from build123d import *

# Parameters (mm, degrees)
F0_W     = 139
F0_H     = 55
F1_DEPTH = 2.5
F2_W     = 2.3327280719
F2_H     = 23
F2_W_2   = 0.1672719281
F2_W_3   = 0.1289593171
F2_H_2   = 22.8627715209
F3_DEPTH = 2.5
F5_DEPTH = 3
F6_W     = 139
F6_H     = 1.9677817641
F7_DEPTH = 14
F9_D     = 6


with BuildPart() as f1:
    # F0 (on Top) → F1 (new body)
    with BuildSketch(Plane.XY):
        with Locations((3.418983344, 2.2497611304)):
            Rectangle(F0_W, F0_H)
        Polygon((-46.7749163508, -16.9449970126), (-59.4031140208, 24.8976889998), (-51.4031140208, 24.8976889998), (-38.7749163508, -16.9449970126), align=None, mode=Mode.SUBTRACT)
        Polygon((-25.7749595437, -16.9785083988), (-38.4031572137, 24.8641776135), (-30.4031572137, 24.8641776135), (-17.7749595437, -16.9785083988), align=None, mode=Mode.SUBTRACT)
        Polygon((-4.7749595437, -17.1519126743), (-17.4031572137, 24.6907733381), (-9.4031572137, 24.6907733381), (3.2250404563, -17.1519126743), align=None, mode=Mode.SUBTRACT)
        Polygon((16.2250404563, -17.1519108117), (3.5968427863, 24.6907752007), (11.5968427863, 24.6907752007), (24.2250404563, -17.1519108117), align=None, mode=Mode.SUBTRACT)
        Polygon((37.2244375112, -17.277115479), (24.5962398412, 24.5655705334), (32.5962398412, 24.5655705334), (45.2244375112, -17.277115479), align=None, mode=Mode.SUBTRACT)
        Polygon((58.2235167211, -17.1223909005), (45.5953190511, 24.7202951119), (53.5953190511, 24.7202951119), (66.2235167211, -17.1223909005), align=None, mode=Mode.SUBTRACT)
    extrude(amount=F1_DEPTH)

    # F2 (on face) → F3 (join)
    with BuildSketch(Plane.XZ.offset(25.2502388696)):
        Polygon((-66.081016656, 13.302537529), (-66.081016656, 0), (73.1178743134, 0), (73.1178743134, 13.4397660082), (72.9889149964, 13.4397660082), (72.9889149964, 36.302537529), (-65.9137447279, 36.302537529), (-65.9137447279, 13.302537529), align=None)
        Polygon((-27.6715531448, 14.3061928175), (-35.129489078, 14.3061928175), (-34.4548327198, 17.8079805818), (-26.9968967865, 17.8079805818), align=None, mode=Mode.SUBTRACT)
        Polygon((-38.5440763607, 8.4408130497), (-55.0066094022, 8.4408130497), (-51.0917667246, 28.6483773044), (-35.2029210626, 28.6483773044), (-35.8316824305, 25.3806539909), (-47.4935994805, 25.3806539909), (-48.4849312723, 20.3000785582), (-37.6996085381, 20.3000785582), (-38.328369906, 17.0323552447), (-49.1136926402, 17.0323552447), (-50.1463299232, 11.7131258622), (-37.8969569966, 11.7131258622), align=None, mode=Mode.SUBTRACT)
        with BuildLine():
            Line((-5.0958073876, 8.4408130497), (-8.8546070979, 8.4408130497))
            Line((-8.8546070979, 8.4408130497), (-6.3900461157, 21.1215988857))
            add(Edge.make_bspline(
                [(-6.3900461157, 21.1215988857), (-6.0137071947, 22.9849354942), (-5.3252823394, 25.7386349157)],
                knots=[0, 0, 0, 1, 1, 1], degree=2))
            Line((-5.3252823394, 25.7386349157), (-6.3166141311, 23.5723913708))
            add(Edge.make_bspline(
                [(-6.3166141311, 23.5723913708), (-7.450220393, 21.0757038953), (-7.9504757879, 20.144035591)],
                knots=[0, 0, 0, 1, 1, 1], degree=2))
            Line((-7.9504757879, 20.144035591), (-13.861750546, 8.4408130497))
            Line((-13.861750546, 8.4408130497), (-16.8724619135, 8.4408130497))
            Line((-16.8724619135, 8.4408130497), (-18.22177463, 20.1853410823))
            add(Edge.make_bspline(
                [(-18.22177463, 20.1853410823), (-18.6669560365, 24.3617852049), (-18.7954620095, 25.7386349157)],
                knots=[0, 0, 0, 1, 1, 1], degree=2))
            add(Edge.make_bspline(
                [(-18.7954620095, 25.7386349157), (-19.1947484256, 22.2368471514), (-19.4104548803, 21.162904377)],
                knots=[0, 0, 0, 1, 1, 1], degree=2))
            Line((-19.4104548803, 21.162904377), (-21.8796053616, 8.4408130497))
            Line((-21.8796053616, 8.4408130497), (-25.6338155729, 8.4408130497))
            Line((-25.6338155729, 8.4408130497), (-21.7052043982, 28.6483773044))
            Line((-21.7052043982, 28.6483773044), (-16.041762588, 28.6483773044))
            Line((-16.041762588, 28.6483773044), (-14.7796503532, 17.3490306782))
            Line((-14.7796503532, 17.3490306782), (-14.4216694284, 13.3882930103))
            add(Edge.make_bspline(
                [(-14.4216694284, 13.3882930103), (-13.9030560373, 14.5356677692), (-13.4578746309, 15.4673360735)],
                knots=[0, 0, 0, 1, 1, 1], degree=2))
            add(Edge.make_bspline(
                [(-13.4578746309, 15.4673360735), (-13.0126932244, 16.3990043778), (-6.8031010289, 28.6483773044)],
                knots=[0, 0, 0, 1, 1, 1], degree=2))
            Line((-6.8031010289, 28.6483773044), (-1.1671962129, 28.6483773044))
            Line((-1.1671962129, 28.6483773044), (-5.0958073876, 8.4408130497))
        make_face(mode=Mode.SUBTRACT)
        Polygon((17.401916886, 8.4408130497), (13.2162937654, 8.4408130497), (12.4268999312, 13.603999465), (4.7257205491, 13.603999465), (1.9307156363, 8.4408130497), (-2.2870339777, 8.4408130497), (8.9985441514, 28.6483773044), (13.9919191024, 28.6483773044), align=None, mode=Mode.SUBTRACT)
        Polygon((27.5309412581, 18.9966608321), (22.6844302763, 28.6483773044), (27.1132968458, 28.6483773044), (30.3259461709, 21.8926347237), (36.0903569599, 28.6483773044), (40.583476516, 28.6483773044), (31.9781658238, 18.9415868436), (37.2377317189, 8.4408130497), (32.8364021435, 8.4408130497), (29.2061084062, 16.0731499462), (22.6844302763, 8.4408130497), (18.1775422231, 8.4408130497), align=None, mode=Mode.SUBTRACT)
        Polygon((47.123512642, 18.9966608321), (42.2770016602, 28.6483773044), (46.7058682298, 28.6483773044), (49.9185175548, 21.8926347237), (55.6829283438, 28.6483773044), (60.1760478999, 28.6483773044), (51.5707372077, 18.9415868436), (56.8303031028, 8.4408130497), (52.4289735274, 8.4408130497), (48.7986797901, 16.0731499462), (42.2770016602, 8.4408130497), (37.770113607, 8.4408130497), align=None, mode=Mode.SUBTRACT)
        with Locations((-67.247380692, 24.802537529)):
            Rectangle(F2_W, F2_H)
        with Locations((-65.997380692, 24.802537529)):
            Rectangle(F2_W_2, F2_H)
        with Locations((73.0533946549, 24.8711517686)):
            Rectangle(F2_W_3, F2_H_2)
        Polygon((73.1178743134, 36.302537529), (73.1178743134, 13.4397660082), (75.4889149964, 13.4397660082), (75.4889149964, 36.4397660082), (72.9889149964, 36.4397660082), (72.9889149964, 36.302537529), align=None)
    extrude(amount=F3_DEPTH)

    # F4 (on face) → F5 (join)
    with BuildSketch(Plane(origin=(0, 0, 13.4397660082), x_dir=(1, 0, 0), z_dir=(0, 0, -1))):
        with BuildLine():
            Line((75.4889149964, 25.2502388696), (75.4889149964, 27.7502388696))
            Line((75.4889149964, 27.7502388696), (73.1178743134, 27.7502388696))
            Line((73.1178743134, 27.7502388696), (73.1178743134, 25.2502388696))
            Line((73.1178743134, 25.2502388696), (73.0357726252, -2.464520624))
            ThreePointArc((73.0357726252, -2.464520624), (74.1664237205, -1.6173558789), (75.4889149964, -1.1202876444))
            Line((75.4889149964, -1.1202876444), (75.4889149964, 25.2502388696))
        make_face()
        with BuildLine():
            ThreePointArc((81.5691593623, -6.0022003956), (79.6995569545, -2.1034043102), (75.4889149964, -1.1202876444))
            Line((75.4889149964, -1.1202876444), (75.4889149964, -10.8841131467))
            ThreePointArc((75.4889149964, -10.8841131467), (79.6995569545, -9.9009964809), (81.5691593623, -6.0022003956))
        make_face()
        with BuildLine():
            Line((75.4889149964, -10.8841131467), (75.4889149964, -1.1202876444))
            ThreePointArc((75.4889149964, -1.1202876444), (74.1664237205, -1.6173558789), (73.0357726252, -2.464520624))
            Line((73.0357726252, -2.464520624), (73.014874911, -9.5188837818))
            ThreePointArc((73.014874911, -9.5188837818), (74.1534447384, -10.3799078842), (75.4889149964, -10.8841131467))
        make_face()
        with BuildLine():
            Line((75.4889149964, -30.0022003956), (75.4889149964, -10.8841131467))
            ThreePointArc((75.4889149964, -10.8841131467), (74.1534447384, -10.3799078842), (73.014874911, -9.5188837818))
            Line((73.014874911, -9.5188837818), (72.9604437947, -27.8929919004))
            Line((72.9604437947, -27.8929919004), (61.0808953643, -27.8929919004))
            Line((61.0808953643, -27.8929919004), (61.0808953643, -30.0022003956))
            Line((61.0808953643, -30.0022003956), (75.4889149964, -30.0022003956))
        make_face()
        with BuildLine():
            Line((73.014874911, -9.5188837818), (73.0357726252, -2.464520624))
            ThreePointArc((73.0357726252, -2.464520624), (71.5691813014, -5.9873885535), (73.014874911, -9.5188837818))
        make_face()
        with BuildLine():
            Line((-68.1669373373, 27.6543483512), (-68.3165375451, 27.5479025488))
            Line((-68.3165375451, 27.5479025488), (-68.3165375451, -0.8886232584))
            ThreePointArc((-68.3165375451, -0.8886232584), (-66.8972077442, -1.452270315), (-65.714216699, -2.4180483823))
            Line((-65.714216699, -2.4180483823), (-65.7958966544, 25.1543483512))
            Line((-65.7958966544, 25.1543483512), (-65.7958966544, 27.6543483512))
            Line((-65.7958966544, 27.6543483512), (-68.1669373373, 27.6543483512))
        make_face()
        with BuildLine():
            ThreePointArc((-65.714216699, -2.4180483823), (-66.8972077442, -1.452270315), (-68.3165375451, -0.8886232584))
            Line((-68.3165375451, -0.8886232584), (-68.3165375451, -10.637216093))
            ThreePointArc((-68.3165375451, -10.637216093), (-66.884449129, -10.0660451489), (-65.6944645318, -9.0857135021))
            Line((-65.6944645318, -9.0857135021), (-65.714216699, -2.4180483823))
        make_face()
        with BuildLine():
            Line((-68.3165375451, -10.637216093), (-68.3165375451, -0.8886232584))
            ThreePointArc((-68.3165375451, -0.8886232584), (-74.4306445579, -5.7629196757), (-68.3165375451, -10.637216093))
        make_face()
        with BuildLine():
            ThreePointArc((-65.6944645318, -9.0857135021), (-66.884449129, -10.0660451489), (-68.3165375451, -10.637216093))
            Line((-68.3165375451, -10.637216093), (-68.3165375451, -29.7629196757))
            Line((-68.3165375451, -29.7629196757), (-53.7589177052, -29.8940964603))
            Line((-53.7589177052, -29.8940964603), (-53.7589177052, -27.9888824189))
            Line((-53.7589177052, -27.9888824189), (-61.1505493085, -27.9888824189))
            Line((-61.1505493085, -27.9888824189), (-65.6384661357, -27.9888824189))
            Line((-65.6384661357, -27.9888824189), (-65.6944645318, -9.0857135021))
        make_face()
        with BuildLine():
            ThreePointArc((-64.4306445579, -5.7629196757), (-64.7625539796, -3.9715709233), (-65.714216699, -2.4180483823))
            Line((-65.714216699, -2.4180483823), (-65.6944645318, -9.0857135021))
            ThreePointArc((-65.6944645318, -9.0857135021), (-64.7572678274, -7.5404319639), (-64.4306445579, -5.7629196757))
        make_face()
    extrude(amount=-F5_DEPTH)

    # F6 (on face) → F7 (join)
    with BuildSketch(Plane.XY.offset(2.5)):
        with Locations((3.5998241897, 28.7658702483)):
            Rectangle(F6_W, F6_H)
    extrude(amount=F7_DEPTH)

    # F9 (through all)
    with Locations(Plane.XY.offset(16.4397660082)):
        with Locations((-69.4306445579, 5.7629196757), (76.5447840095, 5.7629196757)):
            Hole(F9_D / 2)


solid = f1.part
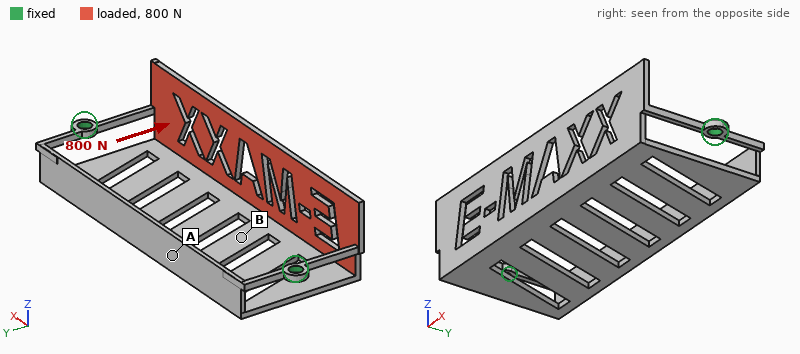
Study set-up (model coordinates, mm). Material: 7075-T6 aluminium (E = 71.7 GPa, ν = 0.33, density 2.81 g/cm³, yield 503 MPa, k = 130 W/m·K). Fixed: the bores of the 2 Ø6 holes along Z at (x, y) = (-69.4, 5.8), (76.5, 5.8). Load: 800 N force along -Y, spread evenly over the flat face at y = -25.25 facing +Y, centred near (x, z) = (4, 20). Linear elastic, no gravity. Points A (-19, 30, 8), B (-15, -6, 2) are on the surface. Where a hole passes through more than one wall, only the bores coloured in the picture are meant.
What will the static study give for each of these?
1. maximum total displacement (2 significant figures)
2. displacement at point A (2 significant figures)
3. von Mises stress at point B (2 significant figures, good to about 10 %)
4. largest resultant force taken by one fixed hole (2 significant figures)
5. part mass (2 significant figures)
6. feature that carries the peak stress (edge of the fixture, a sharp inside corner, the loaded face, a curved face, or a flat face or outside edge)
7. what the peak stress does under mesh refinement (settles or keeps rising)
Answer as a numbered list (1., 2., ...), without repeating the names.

1. 1.9 mm
2. 0.29 mm
3. 60 MPa
4. 400 N
5. 82 g
6. a sharp inside corner
7. keeps rising
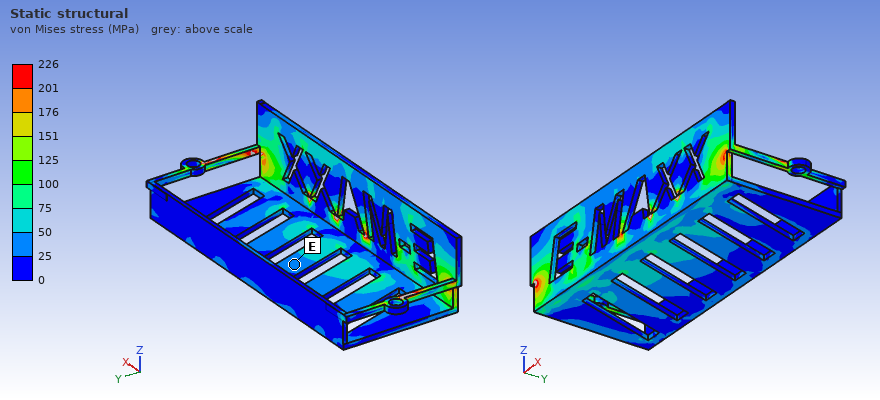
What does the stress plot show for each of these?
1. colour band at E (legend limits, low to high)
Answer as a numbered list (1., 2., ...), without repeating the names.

1. 25 to 50 MPa
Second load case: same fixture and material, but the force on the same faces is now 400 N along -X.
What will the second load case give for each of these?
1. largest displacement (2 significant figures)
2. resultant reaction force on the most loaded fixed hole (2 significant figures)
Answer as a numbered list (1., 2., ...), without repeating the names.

1. 1.0 mm
2. 230 N
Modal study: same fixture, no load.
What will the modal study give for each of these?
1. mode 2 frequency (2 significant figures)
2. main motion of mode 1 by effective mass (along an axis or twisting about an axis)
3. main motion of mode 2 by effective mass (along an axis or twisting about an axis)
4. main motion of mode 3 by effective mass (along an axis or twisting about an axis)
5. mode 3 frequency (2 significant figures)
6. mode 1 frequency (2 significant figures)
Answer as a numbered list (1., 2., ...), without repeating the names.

1. 470 Hz
2. along Z
3. along X
4. along Z
5. 600 Hz
6. 300 Hz
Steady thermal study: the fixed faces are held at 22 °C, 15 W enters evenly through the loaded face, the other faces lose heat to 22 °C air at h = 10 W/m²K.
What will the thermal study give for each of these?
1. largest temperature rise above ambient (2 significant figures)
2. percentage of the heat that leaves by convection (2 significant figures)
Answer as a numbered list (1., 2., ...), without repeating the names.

1. 57 K
2. 65 %
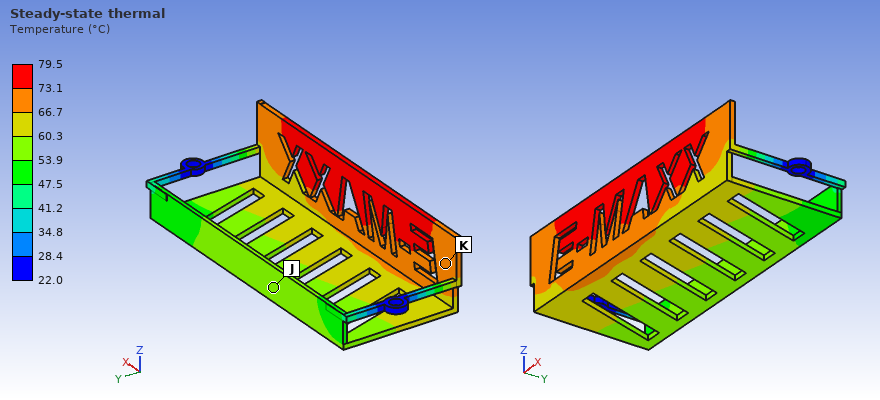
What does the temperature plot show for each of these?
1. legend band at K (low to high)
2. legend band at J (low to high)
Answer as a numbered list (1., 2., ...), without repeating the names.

1. 66.7 to 73.1 °C
2. 53.9 to 60.3 °C
